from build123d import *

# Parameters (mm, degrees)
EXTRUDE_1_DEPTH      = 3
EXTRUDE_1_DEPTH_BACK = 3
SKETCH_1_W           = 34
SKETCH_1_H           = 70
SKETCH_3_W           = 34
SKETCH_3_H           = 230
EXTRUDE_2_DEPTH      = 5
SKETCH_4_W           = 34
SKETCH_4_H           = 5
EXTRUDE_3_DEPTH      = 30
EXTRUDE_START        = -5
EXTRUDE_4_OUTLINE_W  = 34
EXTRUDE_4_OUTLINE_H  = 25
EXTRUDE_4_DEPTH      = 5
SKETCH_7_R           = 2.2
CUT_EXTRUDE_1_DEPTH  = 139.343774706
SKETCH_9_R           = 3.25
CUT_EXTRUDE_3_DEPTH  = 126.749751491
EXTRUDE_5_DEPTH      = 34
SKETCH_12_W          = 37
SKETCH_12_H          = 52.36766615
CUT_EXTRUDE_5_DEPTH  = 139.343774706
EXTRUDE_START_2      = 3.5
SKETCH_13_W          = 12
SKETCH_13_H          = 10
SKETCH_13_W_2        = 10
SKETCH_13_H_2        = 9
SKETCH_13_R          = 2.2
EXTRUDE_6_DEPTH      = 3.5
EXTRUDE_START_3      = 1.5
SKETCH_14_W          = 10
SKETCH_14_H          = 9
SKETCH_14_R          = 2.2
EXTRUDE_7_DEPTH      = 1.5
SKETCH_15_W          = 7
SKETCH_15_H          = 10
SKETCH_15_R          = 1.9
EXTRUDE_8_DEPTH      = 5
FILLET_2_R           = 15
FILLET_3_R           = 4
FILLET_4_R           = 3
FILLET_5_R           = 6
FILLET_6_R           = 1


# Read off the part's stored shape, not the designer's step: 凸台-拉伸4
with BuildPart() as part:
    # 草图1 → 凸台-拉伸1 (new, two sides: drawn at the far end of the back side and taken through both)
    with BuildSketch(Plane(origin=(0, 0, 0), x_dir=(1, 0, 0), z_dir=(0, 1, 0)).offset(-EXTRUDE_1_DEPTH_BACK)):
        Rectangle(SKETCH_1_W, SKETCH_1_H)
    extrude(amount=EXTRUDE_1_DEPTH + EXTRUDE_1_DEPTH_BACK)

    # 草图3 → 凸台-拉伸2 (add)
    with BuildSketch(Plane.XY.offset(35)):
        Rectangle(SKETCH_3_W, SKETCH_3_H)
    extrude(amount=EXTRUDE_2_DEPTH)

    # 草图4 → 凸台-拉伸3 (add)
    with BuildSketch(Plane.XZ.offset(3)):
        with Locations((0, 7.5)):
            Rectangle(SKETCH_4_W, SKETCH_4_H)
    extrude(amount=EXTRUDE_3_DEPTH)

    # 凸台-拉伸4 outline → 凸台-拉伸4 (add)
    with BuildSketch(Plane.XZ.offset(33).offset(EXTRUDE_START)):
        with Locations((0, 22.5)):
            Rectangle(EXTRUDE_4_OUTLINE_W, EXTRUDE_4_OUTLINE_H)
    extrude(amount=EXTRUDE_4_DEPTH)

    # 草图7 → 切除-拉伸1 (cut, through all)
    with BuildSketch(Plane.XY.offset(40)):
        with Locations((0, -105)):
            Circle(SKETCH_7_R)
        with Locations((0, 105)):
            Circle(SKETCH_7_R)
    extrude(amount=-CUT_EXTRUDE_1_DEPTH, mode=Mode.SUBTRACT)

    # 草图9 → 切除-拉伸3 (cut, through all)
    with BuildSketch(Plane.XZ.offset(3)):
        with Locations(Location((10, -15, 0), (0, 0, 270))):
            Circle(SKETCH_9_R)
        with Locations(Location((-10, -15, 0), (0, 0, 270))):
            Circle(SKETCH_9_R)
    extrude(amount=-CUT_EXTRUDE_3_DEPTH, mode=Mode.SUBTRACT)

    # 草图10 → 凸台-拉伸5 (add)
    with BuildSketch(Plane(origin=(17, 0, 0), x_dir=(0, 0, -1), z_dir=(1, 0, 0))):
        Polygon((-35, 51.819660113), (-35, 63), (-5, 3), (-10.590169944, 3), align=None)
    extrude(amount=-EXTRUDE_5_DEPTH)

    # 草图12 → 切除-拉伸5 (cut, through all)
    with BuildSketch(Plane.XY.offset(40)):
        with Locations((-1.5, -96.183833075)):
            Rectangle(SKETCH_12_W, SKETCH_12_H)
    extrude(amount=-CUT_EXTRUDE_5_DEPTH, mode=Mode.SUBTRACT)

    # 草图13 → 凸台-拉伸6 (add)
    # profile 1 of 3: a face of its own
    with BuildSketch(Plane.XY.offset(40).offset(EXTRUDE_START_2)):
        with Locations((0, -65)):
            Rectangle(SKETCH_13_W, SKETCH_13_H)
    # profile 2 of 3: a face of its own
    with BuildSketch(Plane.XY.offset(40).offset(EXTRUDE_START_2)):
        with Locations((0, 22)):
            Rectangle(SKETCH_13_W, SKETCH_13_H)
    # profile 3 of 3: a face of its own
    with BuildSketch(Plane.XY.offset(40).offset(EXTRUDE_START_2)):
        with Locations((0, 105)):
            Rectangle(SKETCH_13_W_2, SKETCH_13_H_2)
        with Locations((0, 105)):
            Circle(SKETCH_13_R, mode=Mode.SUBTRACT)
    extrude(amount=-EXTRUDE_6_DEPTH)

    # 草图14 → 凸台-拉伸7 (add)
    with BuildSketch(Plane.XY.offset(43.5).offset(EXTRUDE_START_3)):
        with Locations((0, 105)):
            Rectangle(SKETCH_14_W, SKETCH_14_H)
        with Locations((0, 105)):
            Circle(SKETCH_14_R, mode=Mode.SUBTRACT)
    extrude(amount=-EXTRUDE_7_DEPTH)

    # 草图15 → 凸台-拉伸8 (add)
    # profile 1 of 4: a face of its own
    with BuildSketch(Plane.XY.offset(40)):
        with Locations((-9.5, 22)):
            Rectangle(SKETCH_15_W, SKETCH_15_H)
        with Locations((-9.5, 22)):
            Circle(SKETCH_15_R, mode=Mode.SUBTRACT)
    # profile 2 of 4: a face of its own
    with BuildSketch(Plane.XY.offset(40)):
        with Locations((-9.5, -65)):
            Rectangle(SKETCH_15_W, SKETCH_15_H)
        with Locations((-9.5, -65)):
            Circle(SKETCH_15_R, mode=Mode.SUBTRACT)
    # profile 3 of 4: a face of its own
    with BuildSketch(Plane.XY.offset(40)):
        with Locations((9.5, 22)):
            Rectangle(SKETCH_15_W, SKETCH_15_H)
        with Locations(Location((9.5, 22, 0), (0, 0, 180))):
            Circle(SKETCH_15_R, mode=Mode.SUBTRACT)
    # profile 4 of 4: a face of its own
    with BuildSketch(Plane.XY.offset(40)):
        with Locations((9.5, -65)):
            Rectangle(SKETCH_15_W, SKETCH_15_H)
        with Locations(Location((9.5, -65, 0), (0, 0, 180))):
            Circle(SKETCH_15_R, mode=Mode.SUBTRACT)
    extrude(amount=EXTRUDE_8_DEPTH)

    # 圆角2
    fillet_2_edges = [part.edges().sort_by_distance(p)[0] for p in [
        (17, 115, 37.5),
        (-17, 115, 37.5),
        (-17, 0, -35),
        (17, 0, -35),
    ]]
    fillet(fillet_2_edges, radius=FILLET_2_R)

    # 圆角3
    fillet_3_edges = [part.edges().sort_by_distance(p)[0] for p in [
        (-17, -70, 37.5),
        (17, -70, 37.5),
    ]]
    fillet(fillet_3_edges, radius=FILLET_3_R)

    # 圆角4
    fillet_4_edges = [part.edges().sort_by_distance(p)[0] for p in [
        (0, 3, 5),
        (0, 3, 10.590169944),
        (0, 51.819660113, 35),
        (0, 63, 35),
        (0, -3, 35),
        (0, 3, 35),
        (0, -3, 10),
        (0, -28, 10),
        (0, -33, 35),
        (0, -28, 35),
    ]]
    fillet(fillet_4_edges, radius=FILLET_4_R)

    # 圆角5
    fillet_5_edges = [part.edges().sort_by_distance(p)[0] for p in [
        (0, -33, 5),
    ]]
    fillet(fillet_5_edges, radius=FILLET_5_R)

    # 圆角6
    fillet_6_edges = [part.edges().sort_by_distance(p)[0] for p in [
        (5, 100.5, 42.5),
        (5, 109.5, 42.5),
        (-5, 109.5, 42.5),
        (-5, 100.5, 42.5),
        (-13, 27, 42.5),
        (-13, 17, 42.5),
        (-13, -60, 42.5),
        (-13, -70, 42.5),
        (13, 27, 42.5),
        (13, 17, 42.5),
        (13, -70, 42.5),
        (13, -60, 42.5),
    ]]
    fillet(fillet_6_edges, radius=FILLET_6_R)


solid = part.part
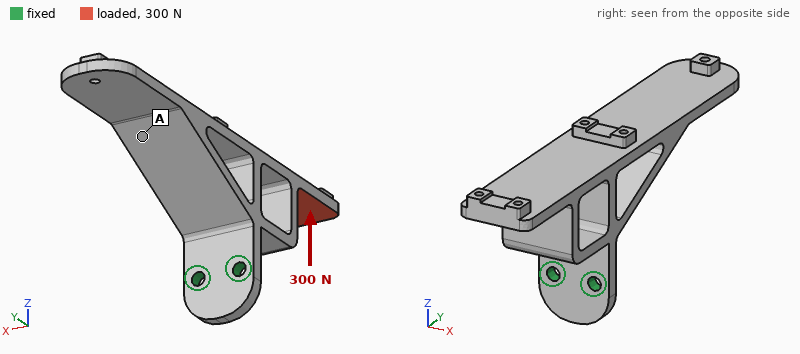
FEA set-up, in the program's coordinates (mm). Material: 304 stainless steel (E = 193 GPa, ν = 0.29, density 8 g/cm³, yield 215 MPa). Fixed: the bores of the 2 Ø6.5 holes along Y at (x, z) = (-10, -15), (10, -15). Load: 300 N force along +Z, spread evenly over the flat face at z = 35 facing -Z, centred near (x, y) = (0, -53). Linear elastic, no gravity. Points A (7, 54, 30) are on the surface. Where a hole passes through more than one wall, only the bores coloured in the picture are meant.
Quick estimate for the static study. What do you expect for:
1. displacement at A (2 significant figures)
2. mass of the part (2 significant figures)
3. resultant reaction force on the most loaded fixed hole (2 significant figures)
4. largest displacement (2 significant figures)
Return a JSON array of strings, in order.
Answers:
["0.18 mm", "540 g", "150 N", "0.35 mm"]
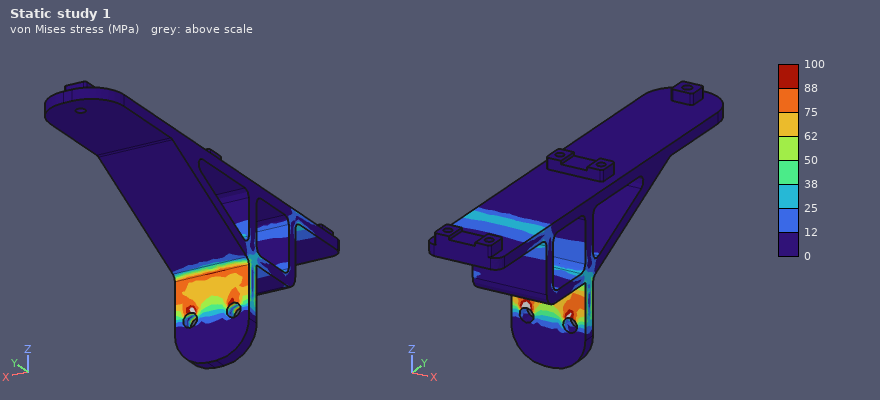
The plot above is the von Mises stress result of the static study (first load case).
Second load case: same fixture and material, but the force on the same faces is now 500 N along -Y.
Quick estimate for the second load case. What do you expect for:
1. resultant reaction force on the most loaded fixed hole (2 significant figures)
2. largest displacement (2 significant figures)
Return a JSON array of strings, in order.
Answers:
["250 N", "0.43 mm"]
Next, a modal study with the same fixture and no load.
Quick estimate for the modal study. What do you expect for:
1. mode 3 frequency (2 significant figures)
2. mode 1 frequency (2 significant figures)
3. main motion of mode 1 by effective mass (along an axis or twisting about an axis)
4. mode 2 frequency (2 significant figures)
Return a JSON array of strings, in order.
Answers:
["1300 Hz", "290 Hz", "along Y", "660 Hz"]
